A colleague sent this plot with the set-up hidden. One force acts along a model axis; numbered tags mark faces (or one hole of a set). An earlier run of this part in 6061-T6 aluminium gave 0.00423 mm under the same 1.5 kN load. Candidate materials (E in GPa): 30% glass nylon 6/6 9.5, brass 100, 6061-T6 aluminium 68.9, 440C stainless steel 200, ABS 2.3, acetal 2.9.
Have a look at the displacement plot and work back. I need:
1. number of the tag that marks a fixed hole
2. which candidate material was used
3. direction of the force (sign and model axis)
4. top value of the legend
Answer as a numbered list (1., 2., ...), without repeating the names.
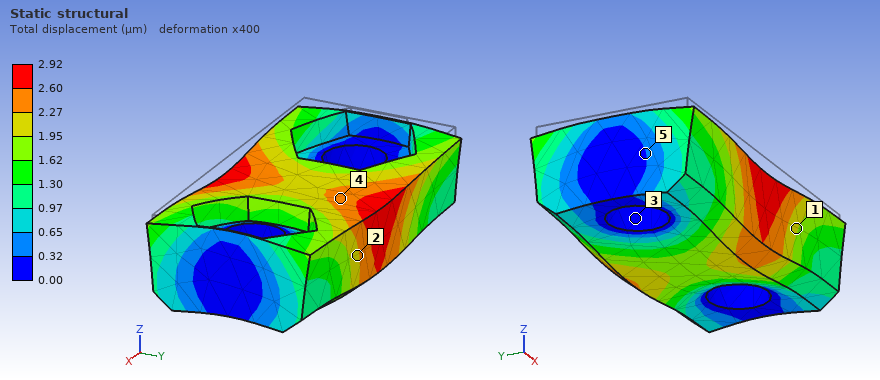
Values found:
1. 3
2. brass
3. -Z
4. 2.92 µm
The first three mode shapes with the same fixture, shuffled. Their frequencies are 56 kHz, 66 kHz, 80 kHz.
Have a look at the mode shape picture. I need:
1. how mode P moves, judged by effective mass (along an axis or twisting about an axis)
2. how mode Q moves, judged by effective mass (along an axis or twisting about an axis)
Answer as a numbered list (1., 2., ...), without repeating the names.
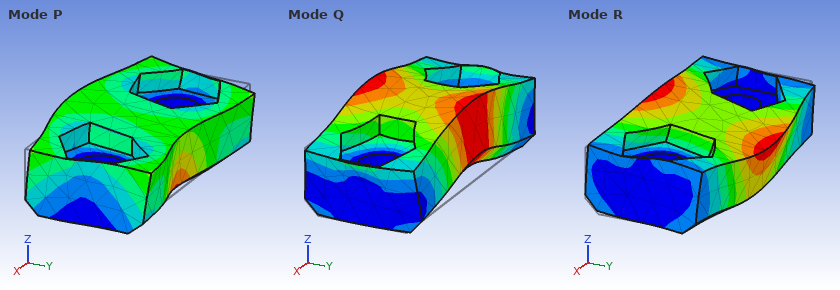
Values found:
1. along Y
2. along Z
